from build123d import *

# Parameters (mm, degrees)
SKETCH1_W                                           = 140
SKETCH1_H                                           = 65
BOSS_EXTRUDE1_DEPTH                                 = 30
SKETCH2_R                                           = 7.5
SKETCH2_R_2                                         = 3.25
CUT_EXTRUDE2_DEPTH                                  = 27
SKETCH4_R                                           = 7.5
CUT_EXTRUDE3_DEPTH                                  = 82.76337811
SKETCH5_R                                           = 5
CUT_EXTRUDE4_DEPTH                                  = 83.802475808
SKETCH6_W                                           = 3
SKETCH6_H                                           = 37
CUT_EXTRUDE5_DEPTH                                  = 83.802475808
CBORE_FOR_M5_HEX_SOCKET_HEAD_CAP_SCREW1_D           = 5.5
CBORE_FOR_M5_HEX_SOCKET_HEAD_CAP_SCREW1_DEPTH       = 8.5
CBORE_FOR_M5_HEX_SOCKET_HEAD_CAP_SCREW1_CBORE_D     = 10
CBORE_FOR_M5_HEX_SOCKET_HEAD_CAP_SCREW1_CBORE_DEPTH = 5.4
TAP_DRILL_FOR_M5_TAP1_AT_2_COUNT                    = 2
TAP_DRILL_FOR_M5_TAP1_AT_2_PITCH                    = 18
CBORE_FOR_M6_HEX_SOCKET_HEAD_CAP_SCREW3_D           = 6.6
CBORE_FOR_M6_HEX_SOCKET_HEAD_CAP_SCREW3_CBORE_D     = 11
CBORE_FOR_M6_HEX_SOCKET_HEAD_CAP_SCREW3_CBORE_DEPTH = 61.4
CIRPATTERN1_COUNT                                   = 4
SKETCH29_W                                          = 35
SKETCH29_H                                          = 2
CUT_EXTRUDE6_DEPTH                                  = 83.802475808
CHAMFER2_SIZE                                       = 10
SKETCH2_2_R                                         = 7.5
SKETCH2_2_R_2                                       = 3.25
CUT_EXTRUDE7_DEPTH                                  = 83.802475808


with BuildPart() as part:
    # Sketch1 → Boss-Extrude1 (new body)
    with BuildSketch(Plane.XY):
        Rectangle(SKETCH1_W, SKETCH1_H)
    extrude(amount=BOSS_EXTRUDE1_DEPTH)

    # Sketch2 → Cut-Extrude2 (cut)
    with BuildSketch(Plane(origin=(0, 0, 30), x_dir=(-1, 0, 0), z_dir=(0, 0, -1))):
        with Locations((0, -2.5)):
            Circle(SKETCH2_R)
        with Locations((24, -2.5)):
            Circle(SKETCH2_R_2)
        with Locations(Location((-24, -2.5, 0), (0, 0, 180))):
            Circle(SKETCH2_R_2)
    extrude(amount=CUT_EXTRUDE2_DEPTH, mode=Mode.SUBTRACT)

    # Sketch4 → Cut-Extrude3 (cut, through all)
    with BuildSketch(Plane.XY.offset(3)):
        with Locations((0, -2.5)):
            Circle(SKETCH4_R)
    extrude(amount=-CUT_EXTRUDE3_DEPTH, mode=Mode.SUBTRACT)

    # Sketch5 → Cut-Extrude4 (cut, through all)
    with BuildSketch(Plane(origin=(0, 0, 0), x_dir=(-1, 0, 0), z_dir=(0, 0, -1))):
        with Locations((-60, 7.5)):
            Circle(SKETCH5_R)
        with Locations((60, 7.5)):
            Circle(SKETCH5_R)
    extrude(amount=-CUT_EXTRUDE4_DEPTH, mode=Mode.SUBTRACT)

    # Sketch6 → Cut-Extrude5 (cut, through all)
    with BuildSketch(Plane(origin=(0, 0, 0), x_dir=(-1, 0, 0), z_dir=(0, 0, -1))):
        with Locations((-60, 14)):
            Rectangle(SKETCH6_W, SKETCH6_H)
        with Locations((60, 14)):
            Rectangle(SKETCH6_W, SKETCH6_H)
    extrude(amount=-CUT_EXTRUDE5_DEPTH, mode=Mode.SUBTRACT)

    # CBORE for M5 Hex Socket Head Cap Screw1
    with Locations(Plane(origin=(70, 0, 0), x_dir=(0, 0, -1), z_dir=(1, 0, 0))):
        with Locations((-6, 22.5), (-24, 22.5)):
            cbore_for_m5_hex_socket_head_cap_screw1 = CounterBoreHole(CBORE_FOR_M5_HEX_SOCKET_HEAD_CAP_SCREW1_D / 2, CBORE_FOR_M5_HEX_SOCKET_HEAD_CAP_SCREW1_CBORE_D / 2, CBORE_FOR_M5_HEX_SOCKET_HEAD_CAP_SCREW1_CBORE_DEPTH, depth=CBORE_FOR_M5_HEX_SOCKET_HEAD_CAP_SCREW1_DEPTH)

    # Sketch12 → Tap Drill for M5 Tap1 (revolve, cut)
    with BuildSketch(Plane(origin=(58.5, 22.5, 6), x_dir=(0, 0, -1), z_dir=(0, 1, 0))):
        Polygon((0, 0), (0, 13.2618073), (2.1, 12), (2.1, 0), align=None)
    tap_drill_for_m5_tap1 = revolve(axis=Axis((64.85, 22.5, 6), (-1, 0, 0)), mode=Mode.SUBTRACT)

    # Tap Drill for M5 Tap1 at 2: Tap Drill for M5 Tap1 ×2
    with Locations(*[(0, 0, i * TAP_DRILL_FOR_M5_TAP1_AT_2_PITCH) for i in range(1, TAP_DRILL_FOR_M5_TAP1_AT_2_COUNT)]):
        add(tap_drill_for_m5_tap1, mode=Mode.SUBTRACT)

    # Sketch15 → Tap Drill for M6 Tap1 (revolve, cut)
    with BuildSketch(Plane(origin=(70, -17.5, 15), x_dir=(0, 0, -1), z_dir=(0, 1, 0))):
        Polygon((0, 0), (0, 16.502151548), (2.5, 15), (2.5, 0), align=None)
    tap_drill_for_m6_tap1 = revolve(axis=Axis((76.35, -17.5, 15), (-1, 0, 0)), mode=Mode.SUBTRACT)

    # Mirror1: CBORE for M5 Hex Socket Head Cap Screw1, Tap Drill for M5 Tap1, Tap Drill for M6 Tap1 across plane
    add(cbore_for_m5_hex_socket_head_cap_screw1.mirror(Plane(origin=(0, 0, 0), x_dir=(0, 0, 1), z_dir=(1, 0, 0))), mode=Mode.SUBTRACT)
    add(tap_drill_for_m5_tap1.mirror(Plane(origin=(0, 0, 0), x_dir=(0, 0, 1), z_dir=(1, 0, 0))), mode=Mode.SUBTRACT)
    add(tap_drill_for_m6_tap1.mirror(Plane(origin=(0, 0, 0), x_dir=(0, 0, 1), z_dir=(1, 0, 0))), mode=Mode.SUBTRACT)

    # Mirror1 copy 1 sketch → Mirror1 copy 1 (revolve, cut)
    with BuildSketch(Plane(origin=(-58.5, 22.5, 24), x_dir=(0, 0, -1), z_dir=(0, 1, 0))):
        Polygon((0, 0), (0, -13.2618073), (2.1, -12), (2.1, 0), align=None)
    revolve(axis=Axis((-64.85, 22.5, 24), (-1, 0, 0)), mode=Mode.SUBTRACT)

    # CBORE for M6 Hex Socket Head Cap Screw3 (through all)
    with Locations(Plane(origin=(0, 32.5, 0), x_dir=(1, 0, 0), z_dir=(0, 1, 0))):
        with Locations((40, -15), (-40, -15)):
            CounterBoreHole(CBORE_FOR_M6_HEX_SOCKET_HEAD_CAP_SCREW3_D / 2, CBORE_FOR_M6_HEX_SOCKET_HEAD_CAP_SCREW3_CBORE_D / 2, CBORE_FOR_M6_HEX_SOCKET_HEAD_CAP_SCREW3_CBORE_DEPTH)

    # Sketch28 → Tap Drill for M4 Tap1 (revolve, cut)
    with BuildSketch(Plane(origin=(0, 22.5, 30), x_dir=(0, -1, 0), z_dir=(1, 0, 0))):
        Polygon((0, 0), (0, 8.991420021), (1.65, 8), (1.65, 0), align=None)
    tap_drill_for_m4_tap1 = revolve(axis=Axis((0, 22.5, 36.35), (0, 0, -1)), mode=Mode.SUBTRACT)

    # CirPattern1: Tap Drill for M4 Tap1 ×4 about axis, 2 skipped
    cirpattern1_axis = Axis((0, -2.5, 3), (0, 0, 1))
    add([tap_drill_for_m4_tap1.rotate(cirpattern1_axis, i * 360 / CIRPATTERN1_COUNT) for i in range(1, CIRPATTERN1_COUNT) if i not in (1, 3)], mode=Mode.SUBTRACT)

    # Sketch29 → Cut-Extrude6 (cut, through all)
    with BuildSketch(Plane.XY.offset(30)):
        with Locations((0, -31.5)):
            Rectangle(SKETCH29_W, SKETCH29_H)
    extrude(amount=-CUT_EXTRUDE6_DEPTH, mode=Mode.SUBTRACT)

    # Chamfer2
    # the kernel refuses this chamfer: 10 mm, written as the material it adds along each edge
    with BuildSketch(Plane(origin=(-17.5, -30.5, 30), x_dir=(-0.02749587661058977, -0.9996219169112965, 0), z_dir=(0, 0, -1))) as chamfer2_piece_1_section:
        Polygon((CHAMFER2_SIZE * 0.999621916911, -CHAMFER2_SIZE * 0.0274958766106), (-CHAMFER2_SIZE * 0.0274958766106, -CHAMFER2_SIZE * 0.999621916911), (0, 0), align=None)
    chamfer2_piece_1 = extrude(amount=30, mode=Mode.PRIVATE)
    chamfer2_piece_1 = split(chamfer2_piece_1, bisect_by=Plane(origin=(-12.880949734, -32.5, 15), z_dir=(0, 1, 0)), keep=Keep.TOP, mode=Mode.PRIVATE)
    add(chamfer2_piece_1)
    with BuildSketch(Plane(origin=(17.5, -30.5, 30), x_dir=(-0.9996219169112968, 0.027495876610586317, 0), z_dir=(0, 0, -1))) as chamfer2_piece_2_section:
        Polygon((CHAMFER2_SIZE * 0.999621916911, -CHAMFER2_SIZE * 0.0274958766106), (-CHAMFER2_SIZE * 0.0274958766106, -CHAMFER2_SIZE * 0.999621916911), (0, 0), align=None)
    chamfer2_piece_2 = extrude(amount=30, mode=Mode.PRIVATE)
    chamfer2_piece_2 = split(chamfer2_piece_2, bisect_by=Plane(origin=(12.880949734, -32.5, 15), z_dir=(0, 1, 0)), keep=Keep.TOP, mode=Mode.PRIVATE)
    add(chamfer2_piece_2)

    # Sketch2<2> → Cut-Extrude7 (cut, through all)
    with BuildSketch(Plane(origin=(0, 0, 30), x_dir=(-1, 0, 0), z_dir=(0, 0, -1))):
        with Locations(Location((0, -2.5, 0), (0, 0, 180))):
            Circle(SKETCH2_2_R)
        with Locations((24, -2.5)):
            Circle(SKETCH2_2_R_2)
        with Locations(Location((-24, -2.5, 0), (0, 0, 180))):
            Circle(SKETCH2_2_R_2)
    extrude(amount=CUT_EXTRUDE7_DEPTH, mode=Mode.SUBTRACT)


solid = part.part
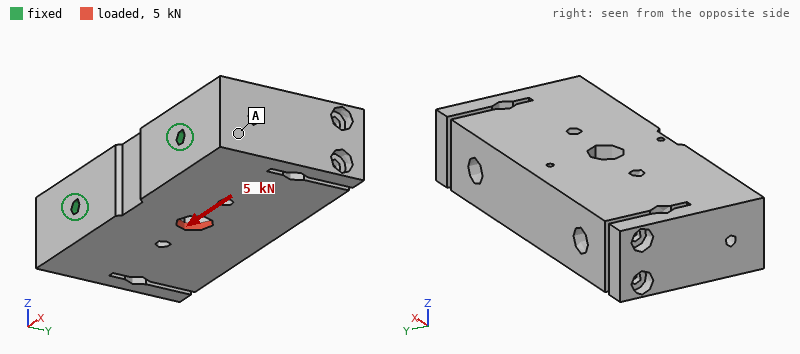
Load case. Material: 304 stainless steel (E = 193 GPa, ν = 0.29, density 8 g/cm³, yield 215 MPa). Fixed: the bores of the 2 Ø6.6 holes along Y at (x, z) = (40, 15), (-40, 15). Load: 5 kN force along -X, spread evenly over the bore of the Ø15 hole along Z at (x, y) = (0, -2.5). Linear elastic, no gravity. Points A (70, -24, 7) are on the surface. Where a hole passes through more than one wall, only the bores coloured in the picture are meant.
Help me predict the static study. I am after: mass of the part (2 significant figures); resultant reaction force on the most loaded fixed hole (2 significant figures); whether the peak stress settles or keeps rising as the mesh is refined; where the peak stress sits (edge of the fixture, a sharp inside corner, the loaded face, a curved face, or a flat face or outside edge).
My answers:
1.9 kg
3.2 kN
keeps rising
edge of the fixture
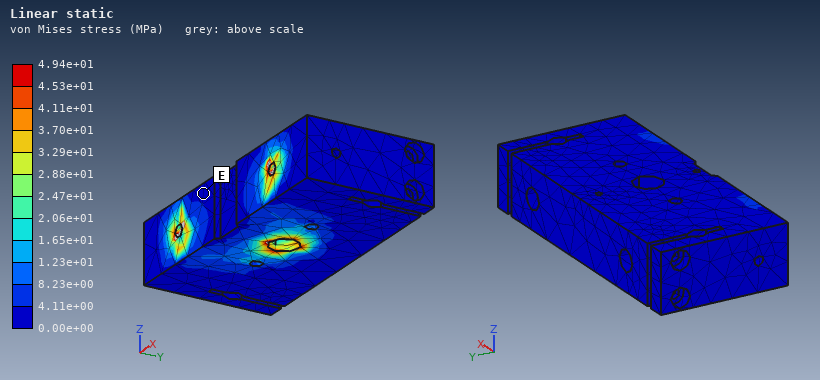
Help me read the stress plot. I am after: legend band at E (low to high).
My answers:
0.00e+00 to 4.11e+00 MPa
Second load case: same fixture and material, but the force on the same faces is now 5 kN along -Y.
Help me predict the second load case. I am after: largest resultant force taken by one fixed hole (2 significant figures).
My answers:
2.6 kN
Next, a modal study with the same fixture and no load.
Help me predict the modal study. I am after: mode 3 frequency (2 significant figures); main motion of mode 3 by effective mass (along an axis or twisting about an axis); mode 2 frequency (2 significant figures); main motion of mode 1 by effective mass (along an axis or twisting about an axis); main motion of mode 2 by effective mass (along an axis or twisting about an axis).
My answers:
3400 Hz
twisting about Y
3200 Hz
along Z
along X
